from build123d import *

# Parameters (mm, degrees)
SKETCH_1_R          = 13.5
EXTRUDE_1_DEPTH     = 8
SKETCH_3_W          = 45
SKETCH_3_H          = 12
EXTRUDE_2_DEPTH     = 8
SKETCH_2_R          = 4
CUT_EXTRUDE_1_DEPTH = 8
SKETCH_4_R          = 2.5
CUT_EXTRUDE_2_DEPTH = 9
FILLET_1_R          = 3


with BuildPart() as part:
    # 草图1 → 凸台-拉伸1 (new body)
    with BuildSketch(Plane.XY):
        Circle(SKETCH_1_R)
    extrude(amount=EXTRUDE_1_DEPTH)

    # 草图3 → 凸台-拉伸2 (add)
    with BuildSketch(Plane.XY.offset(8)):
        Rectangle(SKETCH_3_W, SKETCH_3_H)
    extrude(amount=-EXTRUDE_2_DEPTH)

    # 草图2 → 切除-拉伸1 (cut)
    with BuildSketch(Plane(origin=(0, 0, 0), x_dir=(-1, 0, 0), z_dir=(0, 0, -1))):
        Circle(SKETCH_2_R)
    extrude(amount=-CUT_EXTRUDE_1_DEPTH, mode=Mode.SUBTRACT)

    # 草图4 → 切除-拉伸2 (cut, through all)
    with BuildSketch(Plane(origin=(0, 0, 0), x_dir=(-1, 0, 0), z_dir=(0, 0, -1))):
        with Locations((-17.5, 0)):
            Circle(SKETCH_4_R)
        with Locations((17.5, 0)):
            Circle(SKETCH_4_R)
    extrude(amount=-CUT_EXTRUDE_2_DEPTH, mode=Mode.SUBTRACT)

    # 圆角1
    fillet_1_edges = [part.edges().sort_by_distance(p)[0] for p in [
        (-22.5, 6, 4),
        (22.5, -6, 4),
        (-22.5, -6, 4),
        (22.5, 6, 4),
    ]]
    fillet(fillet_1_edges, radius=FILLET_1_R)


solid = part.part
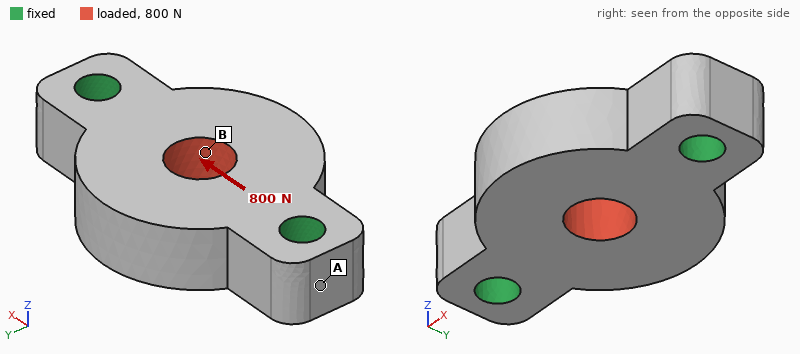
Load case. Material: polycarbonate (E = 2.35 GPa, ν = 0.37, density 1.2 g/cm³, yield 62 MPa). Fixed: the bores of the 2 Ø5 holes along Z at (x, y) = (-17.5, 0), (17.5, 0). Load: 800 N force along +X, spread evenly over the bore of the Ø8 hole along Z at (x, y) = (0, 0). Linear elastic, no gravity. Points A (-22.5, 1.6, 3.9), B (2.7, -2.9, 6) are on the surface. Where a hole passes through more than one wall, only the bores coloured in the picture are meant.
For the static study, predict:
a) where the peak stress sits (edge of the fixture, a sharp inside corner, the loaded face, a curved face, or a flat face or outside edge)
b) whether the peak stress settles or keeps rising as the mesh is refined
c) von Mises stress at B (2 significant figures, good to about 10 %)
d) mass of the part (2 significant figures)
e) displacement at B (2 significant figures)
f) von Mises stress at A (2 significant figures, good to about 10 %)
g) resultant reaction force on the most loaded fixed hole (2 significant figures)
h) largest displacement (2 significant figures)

edge of the fixture
keeps rising
5.7 MPa
6.7 g
26 µm
1.5 MPa
400 N
28 µm
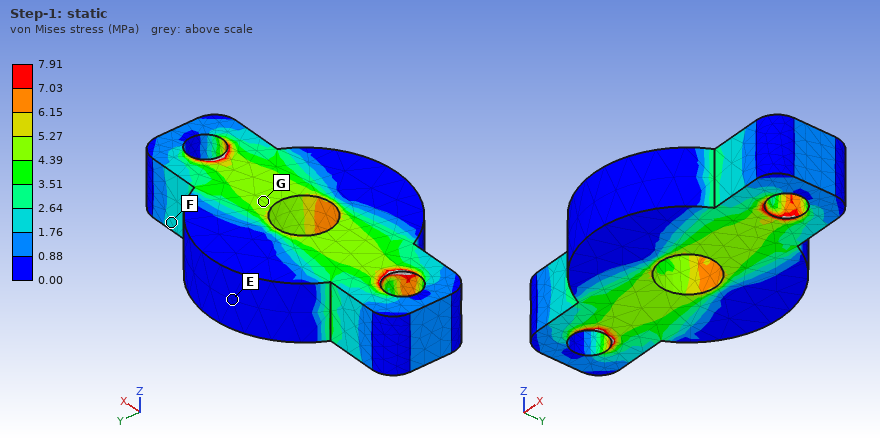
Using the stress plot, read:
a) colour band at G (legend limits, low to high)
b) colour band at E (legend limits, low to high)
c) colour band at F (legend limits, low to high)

4.39 to 5.27 MPa
0.00 to 0.88 MPa
1.76 to 2.64 MPa
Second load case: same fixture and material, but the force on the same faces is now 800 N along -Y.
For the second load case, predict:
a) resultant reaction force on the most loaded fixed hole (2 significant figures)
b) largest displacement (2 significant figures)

400 N
73 µm
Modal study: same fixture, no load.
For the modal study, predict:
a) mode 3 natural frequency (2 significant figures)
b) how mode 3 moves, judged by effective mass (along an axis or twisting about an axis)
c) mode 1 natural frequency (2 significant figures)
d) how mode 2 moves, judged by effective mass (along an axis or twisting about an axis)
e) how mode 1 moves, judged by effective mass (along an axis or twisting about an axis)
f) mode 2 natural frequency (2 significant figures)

9100 Hz
along Y
5100 Hz
along Z
twisting about X
6000 Hz
